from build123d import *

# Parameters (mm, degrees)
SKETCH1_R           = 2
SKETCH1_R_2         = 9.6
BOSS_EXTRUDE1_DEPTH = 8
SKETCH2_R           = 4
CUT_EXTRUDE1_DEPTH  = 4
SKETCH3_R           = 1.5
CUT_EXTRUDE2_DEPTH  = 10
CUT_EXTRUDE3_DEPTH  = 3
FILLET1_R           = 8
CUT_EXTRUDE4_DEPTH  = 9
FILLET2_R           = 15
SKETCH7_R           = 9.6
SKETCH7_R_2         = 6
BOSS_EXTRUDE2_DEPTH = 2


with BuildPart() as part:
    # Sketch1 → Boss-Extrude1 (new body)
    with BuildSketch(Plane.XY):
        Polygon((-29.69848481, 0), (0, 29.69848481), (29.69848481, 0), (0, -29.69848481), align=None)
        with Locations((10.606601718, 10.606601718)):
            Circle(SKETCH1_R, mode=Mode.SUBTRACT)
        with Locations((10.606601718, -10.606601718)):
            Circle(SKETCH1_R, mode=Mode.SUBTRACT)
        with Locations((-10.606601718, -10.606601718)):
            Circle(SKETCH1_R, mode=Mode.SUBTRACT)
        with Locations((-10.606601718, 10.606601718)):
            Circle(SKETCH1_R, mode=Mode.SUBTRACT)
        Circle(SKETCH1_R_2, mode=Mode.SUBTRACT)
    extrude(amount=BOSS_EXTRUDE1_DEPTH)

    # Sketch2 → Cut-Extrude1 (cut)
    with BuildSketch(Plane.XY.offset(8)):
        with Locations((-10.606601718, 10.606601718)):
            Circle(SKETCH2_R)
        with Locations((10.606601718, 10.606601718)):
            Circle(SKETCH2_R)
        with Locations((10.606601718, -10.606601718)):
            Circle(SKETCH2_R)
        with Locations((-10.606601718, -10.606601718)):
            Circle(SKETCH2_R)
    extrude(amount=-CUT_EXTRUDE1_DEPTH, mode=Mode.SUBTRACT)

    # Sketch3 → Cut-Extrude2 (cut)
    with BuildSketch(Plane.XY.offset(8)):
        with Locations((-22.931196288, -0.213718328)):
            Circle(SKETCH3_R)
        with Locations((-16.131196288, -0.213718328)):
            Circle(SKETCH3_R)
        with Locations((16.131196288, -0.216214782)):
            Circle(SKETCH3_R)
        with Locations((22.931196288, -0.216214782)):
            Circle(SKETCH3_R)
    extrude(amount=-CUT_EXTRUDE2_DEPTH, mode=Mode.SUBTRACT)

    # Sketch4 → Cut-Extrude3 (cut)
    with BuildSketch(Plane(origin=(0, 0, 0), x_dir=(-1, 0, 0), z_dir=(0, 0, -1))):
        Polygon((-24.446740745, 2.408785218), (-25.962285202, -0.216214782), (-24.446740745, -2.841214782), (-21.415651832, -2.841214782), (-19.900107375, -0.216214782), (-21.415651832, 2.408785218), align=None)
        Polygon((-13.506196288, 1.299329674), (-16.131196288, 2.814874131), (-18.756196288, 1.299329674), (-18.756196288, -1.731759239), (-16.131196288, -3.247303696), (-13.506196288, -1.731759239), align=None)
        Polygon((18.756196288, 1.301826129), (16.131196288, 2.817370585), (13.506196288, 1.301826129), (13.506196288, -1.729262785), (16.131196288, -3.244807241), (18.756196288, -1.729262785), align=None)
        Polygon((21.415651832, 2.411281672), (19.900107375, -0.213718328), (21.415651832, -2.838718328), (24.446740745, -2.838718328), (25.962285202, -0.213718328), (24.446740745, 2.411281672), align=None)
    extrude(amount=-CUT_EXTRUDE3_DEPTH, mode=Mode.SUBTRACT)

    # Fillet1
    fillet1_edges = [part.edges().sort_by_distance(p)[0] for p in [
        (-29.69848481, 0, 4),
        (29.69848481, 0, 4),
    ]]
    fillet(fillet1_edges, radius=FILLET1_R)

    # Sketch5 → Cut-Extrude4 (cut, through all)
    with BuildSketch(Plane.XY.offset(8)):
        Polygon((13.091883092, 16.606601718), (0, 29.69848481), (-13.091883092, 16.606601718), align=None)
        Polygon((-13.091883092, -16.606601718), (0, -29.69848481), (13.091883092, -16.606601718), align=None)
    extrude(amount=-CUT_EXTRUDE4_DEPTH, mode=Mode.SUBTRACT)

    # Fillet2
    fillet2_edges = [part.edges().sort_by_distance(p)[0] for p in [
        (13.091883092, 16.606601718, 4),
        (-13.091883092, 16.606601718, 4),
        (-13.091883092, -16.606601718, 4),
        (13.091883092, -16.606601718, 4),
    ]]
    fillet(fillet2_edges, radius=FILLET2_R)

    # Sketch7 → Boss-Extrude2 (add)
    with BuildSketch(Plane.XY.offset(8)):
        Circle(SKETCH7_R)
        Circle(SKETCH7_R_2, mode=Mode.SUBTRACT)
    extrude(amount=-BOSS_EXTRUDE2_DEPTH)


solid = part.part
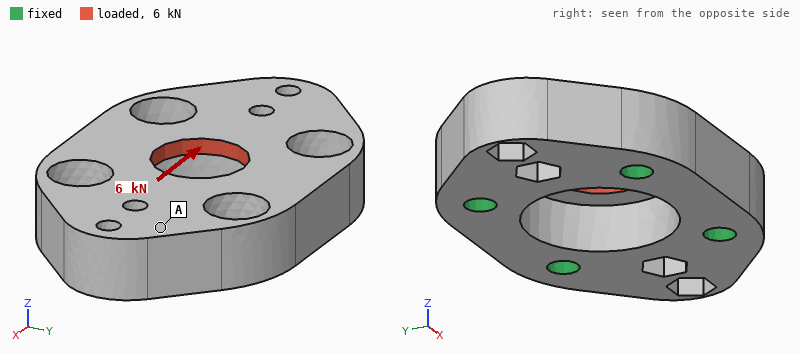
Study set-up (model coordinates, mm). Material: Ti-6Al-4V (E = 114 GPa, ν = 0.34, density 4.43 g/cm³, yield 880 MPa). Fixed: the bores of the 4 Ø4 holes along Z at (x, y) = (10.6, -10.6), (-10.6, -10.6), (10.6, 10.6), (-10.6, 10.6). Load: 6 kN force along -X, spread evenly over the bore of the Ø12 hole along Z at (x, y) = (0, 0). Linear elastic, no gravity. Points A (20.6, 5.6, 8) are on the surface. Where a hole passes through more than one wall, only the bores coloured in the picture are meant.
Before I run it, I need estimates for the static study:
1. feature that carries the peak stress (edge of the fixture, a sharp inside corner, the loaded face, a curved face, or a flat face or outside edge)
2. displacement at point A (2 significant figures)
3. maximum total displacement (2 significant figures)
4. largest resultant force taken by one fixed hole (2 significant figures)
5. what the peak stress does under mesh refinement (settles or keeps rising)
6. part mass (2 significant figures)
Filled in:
a sharp inside corner
11 µm
16 µm
1.6 kN
keeps rising
34 g
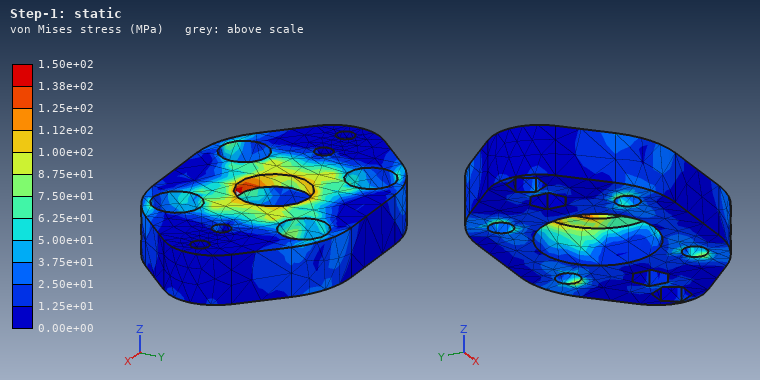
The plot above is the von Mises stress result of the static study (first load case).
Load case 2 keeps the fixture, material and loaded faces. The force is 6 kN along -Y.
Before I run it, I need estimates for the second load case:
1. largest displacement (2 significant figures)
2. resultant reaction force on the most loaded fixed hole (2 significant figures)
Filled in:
16 µm
1.6 kN
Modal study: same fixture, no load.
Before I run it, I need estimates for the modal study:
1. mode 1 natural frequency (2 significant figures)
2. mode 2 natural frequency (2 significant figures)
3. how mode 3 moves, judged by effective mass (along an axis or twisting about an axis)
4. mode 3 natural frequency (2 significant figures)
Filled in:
19 kHz
19 kHz
along Y
42 kHz
